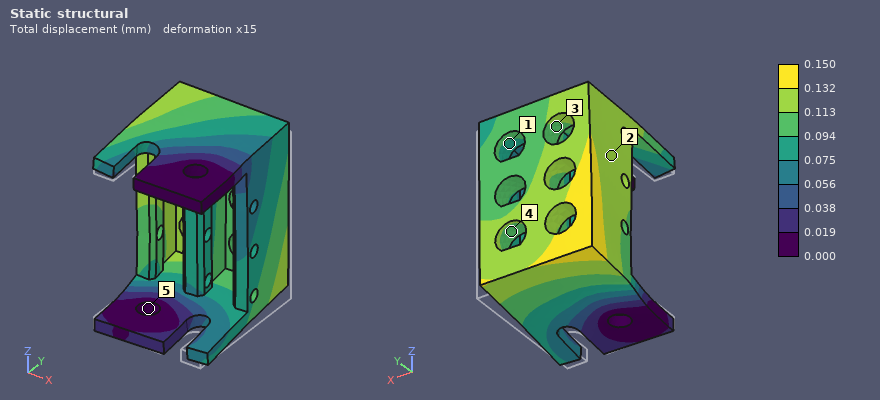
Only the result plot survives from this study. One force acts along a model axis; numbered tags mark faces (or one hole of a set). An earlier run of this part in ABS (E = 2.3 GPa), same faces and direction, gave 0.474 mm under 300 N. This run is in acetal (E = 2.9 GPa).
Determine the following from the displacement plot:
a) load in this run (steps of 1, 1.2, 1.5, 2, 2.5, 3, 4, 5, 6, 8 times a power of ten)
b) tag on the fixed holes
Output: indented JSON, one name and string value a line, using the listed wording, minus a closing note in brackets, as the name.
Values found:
{
  "load in this run": "120 N",
  "tag on the fixed holes": "5"
}
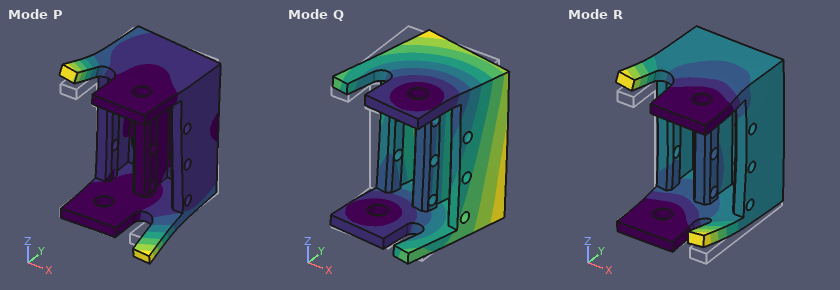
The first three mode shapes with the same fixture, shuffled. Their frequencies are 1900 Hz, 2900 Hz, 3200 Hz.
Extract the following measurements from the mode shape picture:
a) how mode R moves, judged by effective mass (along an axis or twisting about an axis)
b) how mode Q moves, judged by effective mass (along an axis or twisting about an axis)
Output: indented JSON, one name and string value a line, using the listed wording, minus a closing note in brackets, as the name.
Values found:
{
  "how mode R moves, judged by effective mass": "along Z",
  "how mode Q moves, judged by effective mass": "along X"
}
